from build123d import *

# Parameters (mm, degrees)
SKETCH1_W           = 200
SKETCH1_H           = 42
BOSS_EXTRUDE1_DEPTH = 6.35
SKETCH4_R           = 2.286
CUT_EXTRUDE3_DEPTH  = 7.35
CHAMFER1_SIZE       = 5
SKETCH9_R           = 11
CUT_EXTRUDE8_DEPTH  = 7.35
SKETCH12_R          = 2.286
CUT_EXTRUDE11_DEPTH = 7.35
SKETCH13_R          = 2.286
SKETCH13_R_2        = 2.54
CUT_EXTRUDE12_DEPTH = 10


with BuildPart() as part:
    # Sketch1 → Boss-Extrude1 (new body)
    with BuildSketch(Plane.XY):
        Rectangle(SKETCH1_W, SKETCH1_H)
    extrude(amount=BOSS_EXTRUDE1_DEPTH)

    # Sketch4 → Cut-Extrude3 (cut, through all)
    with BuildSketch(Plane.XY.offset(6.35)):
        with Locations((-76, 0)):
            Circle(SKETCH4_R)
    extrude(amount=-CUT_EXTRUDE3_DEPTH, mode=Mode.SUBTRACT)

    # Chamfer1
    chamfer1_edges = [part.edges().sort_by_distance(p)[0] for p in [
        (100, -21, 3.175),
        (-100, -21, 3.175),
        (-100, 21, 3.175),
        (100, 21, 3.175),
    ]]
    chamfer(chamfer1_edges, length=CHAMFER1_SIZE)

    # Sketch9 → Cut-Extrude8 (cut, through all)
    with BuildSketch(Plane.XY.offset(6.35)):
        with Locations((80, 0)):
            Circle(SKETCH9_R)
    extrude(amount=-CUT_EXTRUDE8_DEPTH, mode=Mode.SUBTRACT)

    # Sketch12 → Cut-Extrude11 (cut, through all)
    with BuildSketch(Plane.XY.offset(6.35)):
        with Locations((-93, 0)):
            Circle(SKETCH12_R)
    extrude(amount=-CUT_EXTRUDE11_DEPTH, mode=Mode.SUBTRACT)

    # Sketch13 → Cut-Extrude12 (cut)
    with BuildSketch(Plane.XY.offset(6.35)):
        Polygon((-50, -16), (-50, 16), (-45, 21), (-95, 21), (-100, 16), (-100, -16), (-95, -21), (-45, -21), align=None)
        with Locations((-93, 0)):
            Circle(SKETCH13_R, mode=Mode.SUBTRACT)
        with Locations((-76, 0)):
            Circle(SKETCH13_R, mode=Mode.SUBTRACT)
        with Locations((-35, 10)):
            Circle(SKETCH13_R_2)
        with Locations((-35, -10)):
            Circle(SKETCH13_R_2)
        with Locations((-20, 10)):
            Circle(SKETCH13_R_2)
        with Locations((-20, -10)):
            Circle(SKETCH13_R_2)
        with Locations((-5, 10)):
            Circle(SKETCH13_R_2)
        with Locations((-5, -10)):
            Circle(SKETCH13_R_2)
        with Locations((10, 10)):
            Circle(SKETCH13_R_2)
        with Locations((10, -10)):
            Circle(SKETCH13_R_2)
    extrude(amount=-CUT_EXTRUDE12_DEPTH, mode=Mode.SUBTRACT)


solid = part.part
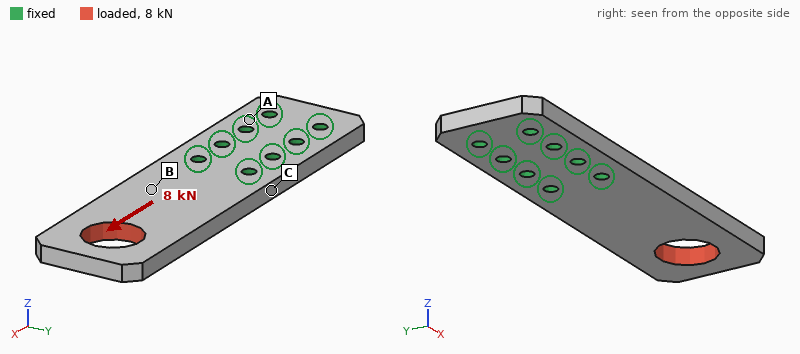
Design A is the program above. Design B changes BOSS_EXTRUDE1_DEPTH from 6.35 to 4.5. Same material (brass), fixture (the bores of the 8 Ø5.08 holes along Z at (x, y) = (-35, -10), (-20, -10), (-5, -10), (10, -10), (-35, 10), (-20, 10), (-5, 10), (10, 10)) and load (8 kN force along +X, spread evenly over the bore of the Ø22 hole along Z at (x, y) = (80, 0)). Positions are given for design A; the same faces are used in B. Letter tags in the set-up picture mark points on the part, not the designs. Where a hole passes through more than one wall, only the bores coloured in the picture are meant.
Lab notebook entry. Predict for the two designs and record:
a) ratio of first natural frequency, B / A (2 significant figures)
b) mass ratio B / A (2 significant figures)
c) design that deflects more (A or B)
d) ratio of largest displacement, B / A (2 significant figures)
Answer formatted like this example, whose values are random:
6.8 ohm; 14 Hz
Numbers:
0.72; 0.71; B; 1.4
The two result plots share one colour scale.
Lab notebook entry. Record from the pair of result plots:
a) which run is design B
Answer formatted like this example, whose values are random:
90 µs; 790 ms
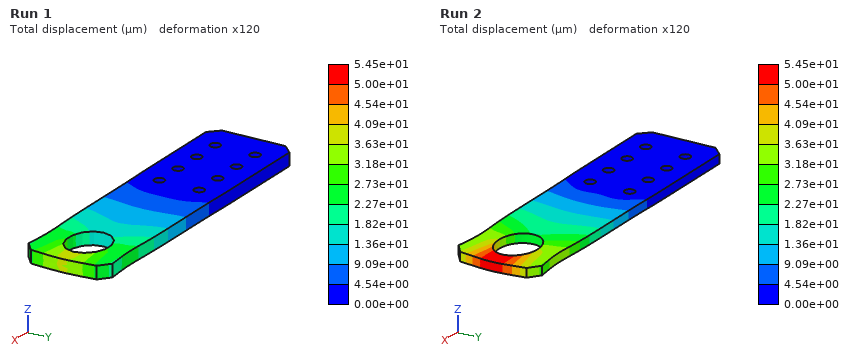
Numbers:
Run 2
